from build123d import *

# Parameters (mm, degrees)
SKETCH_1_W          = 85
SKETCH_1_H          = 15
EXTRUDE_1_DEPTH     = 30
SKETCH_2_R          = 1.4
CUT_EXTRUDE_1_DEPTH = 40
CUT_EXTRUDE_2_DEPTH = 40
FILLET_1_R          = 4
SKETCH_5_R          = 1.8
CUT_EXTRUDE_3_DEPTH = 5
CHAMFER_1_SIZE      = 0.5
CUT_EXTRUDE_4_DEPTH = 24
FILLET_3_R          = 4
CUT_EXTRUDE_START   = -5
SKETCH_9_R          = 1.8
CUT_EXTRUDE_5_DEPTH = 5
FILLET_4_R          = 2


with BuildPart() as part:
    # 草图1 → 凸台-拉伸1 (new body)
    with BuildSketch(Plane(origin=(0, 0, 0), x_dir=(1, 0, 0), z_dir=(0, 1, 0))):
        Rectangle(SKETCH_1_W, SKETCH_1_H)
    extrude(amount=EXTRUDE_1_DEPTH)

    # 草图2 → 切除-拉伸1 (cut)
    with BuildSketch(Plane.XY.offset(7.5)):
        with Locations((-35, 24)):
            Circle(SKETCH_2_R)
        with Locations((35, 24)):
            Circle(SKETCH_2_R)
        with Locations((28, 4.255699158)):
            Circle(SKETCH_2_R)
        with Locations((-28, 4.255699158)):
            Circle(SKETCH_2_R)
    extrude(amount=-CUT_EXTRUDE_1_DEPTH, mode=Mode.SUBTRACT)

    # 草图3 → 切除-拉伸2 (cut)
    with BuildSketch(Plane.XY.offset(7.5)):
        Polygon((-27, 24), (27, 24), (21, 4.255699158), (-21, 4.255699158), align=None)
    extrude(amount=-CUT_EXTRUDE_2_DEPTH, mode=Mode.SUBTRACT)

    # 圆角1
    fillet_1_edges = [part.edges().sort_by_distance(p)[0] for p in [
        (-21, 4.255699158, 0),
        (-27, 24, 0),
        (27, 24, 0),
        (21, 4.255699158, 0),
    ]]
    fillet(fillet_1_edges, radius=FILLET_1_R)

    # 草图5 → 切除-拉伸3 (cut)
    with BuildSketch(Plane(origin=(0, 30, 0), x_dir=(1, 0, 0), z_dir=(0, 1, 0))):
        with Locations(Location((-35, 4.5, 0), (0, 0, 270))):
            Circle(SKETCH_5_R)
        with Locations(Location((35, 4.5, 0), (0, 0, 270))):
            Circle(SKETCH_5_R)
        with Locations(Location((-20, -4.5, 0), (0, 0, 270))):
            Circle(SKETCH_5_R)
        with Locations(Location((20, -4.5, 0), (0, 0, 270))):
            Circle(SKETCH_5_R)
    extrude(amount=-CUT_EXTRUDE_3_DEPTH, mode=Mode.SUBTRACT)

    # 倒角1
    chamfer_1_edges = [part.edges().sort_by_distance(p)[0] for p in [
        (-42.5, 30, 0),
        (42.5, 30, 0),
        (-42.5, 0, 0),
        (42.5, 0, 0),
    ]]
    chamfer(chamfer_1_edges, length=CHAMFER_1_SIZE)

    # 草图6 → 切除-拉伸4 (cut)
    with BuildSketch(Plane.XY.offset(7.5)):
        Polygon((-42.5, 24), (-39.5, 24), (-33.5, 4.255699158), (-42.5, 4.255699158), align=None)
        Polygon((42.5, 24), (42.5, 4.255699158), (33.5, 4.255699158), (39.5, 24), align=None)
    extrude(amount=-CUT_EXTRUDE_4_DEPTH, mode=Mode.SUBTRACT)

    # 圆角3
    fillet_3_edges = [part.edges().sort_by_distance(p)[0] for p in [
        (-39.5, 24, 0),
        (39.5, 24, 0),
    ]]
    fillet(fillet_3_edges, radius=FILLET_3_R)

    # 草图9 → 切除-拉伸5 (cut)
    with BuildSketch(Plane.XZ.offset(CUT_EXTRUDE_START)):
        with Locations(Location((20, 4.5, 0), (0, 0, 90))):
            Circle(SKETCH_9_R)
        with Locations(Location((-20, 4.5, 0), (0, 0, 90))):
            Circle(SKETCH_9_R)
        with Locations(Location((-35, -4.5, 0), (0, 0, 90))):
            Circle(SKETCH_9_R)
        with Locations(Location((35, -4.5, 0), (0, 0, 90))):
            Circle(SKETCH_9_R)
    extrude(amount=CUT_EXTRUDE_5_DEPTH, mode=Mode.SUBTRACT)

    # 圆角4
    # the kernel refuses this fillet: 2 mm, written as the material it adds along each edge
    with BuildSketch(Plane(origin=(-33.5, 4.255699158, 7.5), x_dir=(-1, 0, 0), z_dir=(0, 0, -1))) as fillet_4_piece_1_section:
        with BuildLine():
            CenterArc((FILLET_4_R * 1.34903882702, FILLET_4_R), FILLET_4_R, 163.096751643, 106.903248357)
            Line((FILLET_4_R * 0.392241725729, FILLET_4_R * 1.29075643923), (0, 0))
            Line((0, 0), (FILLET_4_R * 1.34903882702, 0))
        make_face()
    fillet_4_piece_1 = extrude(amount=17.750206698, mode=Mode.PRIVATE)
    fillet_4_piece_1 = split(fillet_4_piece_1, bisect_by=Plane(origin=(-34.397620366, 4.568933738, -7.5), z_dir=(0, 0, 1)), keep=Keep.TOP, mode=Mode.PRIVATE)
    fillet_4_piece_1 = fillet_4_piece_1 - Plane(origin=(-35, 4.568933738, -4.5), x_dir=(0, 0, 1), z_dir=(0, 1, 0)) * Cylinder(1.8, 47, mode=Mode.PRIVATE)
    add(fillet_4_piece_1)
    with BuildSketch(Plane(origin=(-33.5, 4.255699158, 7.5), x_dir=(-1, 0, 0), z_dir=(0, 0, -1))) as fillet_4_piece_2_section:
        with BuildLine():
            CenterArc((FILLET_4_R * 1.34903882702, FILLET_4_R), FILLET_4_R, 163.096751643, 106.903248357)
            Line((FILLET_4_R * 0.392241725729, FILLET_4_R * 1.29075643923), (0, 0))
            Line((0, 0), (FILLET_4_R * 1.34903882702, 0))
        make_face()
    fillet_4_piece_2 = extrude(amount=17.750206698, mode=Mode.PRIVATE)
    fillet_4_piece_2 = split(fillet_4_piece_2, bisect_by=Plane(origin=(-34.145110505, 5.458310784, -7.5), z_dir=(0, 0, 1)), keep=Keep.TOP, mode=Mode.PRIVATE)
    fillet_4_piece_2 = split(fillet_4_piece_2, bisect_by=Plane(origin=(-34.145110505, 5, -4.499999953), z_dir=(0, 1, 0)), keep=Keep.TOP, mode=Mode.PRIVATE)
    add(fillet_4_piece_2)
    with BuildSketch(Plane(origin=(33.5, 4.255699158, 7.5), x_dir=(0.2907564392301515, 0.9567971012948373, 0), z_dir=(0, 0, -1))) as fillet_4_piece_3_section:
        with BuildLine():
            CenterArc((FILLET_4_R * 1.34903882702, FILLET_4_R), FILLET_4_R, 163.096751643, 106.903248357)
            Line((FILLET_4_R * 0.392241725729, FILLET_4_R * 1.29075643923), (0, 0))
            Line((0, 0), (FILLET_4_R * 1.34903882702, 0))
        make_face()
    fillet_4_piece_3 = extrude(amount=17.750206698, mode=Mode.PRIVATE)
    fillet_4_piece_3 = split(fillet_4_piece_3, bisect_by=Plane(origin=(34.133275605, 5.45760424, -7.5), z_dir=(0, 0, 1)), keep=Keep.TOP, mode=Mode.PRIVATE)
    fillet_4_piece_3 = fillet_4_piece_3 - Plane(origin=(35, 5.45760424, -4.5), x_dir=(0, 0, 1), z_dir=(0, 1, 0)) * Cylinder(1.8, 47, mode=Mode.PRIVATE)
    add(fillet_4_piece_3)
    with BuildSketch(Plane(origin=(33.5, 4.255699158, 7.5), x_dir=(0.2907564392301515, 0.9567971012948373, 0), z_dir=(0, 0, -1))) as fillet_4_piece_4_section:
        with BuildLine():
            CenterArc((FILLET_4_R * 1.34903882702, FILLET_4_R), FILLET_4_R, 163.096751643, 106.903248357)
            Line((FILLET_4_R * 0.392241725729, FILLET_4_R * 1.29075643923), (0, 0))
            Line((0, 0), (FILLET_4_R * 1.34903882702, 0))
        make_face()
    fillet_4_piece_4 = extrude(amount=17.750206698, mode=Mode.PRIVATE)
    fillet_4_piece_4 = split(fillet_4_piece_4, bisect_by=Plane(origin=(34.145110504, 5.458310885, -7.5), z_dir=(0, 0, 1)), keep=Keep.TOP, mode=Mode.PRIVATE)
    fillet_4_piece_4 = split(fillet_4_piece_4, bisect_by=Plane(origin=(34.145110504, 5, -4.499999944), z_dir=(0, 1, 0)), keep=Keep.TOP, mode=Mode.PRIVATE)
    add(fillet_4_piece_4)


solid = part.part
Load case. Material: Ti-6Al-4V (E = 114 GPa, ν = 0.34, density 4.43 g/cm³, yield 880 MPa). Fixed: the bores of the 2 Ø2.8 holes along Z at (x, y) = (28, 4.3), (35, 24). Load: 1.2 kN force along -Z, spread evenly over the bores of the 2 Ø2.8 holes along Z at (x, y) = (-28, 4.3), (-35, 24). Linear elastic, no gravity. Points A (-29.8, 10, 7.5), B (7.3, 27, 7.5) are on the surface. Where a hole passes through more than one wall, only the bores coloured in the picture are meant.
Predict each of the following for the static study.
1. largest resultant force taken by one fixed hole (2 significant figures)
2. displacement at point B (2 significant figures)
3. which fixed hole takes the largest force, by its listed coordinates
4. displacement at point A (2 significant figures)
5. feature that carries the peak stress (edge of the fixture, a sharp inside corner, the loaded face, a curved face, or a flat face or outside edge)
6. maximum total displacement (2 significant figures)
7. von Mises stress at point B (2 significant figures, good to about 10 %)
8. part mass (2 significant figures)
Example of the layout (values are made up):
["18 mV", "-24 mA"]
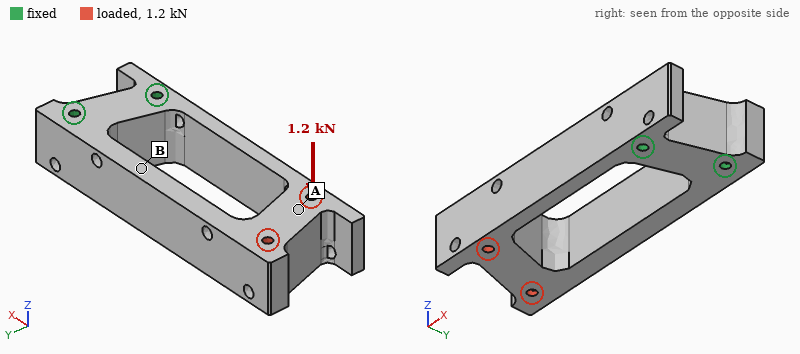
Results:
["980 N", "0.075 mm", "(28, 4.3)", "0.30 mm", "a curved face", "0.40 mm", "110 MPa", "89 g"]
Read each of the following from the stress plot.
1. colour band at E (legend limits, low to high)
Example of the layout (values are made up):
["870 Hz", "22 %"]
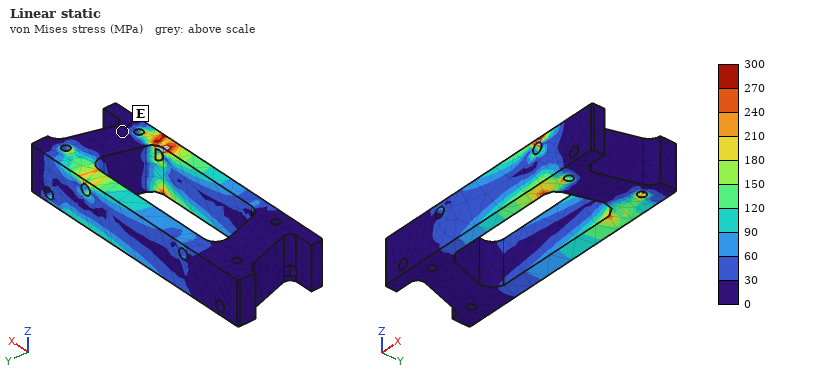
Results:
["0 to 30 MPa"]
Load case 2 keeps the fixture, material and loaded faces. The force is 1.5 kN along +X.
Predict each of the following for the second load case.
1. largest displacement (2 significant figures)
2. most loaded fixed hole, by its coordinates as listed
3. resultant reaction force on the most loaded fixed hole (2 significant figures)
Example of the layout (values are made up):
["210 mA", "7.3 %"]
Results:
["9.0 µm", "(28, 4.3)", "810 N"]
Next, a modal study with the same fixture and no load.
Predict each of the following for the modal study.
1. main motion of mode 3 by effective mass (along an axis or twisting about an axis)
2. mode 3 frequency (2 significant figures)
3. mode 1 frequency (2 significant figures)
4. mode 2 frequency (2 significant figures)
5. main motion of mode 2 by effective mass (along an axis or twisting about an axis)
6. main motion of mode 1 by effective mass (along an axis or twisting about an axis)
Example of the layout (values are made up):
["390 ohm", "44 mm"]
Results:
["twisting about X", "4000 Hz", "1400 Hz", "1700 Hz", "along Z", "along Y"]
